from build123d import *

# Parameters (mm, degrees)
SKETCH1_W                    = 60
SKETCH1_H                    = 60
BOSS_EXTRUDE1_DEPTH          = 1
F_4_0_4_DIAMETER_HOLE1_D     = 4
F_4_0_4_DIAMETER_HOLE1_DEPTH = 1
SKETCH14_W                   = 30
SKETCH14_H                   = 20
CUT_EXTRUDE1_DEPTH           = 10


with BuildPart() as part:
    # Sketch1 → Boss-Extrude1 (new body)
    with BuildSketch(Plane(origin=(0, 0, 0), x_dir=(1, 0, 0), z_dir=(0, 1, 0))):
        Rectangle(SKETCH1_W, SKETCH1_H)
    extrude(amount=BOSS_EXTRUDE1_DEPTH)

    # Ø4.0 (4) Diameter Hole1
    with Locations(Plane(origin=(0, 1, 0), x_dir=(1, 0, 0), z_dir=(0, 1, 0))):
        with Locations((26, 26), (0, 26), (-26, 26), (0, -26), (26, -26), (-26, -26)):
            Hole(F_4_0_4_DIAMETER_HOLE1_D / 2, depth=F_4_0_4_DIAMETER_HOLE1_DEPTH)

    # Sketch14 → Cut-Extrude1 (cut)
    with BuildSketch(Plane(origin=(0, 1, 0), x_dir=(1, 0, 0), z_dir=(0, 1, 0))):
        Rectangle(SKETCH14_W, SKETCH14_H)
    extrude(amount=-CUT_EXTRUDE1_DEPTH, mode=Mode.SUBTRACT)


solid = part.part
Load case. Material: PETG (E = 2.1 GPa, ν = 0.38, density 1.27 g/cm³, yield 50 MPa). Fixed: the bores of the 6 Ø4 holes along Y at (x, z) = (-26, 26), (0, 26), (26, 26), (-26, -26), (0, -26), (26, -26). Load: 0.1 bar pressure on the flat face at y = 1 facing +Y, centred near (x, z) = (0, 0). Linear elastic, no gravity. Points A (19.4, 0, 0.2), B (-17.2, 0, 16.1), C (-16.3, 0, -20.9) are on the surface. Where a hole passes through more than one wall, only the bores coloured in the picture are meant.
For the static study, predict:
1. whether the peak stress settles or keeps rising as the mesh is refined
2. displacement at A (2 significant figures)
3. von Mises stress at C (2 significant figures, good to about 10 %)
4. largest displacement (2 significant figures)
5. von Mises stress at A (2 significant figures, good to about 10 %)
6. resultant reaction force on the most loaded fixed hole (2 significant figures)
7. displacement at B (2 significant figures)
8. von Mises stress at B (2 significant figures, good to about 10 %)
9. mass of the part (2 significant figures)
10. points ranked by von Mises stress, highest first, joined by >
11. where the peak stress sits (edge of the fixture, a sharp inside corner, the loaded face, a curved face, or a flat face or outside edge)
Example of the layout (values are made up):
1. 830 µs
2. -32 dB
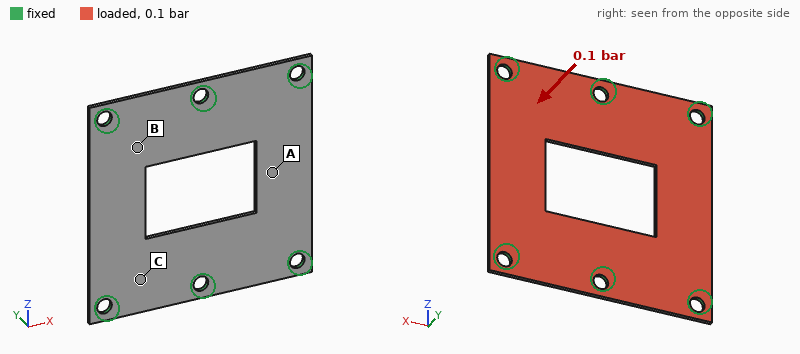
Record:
1. keeps rising
2. 0.88 mm
3. 3.5 MPa
4. 0.93 mm
5. 5.6 MPa
6. 5.8 N
7. 0.36 mm
8. 2.0 MPa
9. 3.7 g
10. A > C > B
11. edge of the fixture
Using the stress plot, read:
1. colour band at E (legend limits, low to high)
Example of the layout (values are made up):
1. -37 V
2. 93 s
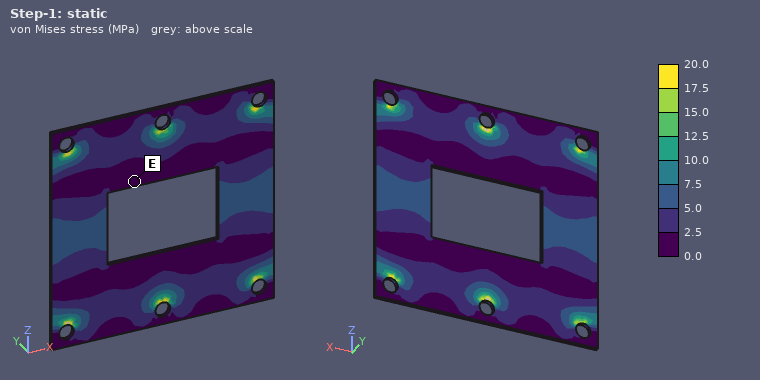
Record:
1. 0.0 to 2.5 MPa
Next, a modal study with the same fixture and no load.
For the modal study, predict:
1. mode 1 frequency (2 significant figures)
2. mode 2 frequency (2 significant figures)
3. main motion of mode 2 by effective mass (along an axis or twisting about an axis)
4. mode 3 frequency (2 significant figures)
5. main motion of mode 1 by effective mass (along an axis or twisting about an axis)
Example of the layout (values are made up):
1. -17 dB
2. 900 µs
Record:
1. 570 Hz
2. 600 Hz
3. twisting about Z
4. 1100 Hz
5. along Y
